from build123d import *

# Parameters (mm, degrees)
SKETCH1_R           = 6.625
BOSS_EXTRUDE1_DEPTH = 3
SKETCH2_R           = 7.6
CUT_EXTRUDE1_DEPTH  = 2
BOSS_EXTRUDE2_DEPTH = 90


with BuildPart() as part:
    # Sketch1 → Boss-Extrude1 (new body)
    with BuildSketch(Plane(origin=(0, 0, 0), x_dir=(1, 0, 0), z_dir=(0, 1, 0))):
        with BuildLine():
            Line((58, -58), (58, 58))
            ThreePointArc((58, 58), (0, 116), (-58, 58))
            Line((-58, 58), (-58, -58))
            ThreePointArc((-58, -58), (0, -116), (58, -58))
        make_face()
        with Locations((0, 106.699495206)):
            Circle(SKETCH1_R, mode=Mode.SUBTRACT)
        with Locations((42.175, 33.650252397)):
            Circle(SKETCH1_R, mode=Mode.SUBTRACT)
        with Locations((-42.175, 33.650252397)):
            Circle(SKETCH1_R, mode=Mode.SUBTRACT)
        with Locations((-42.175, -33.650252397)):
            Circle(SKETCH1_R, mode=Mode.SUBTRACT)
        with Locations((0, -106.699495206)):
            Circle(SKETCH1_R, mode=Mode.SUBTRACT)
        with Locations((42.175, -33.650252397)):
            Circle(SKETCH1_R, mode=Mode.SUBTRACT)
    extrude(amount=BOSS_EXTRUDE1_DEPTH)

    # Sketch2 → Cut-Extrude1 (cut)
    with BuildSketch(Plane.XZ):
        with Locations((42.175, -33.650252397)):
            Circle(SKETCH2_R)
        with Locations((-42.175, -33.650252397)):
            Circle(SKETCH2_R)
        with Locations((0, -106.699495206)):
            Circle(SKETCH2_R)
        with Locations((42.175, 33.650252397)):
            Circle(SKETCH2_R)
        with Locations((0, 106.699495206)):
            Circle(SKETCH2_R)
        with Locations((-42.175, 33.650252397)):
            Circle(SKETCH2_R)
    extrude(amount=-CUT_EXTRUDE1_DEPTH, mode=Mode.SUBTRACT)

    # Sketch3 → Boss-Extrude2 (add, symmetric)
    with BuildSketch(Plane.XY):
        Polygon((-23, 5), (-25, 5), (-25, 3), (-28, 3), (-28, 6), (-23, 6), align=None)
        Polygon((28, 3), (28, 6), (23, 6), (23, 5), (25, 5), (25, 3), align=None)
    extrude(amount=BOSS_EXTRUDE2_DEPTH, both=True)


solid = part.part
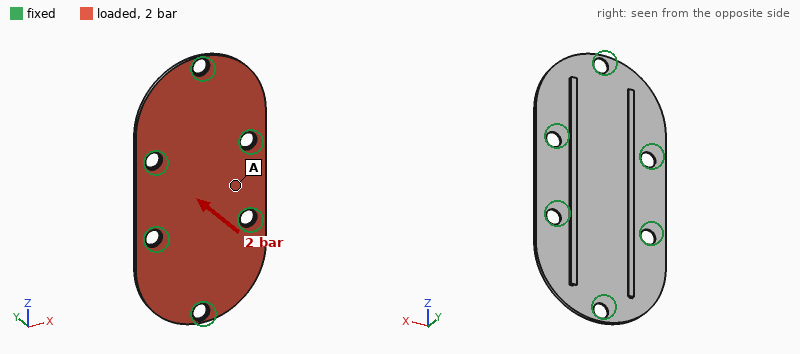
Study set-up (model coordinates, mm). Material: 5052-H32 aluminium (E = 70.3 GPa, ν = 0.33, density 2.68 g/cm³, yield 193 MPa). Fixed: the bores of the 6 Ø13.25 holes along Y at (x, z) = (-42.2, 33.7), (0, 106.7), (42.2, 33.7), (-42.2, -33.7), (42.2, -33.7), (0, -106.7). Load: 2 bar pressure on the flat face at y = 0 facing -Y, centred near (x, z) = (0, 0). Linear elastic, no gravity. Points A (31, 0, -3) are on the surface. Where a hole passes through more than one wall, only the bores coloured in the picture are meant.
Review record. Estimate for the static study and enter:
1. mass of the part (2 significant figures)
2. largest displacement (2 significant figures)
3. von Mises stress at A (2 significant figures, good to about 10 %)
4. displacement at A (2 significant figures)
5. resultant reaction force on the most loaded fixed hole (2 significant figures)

200 g
0.31 mm
25 MPa
0.077 mm
1.2 kN
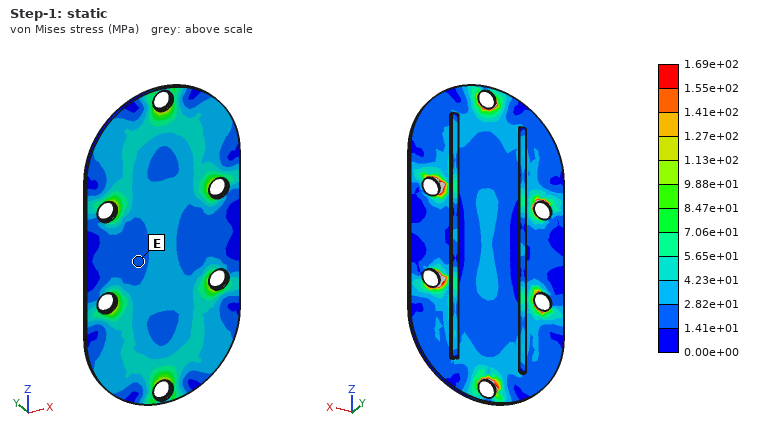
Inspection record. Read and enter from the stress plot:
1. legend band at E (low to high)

1.41e+01 to 2.82e+01 MPa
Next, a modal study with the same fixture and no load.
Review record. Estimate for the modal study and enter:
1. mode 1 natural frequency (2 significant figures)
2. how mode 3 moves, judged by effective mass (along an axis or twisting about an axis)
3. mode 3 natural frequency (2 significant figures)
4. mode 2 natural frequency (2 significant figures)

1700 Hz
along Y
1800 Hz
1700 Hz
